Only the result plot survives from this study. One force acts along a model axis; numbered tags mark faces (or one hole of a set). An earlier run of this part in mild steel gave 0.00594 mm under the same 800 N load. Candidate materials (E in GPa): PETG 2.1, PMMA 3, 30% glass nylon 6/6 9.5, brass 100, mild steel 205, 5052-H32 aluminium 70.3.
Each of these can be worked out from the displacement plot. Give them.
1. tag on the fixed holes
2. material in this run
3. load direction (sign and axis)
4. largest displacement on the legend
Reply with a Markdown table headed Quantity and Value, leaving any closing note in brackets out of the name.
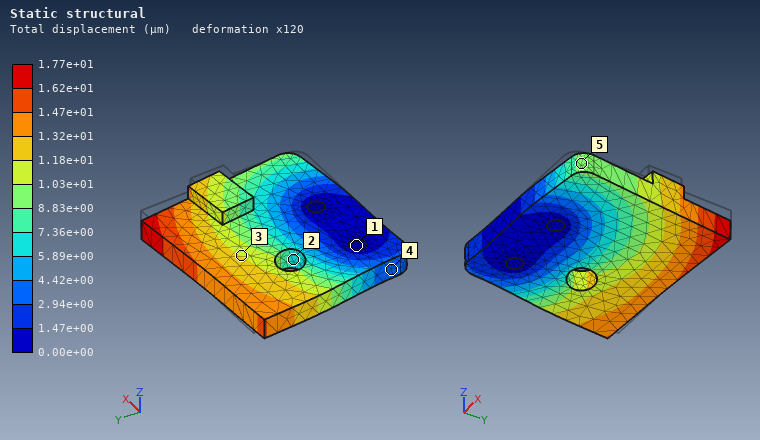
| Quantity | Value |
|---|---|
| tag on the fixed holes | 1 |
| material in this run | 5052-H32 aluminium |
| load direction | -X |
| largest displacement on the legend | 1.77e+01 µm |
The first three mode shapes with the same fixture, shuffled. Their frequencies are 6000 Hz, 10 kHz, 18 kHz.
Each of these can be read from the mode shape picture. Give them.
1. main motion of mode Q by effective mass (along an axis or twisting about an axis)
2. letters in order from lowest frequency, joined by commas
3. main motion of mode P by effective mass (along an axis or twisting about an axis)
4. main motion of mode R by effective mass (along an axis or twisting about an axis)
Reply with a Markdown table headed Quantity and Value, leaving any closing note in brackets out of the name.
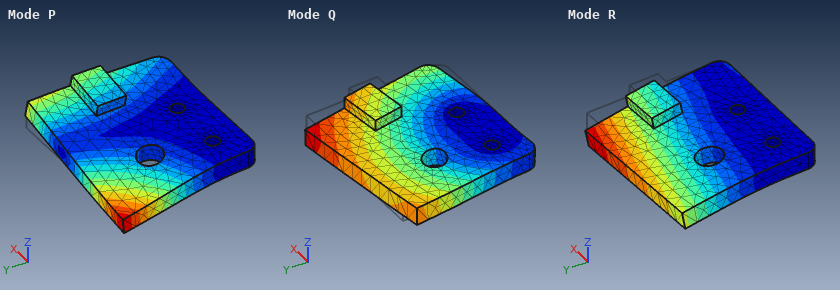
| Quantity | Value |
|---|---|
| main motion of mode Q by effective mass | along X |
| letters in order from lowest frequency, joined by commas | R, P, Q |
| main motion of mode P by effective mass | twisting about Y |
| main motion of mode R by effective mass | along Z |
